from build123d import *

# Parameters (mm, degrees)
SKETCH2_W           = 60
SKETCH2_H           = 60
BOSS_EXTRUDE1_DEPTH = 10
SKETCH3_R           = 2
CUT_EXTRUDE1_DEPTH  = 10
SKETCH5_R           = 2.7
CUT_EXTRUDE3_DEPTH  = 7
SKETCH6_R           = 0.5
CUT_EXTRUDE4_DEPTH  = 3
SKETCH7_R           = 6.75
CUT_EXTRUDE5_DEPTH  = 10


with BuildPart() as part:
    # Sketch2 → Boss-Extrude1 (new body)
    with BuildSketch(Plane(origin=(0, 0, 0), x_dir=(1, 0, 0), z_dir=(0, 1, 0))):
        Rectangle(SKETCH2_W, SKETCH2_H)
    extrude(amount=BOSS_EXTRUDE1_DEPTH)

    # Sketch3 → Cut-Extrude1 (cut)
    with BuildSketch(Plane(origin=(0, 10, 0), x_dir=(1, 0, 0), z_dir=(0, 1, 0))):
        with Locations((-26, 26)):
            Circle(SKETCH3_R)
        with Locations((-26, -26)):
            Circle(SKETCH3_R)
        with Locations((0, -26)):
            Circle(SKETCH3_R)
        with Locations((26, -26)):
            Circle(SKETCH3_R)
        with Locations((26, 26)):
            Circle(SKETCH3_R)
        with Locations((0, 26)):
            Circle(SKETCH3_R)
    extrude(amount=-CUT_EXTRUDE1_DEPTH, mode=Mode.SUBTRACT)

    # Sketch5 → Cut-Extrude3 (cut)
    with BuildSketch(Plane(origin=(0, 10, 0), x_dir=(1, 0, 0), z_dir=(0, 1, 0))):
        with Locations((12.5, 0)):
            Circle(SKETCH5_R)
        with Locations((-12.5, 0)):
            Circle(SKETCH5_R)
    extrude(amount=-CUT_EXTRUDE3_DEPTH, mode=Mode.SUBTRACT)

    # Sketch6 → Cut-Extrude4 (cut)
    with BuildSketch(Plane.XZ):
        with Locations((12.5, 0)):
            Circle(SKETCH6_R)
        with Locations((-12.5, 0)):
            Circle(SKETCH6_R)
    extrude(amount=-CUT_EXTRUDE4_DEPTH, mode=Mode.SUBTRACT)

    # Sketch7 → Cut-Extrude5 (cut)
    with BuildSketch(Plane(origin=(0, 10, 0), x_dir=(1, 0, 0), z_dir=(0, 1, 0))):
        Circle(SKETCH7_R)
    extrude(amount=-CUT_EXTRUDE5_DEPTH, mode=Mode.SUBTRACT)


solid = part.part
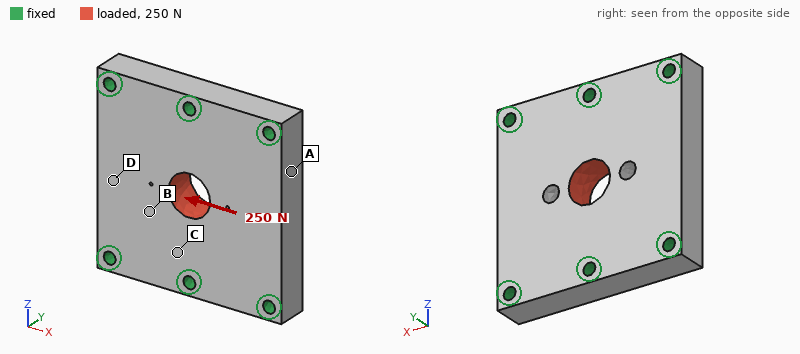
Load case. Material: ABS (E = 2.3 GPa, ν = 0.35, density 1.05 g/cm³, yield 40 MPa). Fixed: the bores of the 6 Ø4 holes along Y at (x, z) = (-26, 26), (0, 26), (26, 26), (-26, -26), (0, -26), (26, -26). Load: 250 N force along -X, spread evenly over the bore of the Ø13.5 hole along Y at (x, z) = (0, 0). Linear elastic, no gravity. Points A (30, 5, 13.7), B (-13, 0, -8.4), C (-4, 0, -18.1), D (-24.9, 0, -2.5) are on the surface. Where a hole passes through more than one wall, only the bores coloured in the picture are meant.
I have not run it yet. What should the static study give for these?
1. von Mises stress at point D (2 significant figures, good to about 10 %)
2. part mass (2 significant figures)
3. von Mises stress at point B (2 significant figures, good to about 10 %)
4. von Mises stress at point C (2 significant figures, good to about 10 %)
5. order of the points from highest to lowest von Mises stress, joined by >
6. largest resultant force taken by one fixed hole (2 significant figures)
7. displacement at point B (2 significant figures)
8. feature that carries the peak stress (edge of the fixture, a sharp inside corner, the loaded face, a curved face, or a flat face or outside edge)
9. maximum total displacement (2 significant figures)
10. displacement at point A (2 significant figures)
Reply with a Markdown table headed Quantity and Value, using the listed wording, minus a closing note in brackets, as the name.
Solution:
| Quantity | Value |
|---|---|
| von Mises stress at point D | 0.16 MPa |
| part mass | 35 g |
| von Mises stress at point B | 0.45 MPa |
| von Mises stress at point C | 0.37 MPa |
| order of the points from highest to lowest von Mises stress, joined by > | B > C > D > A |
| largest resultant force taken by one fixed hole | 54 N |
| displacement at point B | 5.2 µm |
| feature that carries the peak stress | a curved face |
| maximum total displacement | 9.2 µm |
| displacement at point A | 3.6 µm |
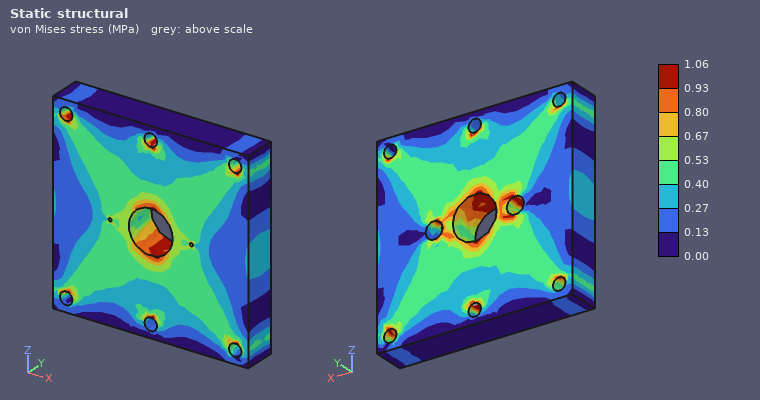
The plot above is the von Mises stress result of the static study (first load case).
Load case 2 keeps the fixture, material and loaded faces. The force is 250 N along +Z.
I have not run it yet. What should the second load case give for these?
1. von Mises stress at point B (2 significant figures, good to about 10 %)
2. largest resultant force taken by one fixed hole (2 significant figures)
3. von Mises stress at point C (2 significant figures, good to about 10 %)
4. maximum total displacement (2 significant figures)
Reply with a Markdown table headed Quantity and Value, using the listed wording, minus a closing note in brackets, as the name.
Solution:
| Quantity | Value |
|---|---|
| von Mises stress at point B | 0.25 MPa |
| largest resultant force taken by one fixed hole | 71 N |
| von Mises stress at point C | 0.45 MPa |
| maximum total displacement | 5.1 µm |
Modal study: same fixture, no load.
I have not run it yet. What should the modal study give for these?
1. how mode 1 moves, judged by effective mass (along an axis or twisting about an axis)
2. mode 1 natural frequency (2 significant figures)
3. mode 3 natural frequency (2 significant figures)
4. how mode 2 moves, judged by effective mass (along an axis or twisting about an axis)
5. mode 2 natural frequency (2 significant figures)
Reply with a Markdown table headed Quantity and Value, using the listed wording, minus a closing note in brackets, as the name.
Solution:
| Quantity | Value |
|---|---|
| how mode 1 moves, judged by effective mass | along Y |
| mode 1 natural frequency | 4100 Hz |
| mode 3 natural frequency | 7400 Hz |
| how mode 2 moves, judged by effective mass | twisting about Z |
| mode 2 natural frequency | 4900 Hz |
